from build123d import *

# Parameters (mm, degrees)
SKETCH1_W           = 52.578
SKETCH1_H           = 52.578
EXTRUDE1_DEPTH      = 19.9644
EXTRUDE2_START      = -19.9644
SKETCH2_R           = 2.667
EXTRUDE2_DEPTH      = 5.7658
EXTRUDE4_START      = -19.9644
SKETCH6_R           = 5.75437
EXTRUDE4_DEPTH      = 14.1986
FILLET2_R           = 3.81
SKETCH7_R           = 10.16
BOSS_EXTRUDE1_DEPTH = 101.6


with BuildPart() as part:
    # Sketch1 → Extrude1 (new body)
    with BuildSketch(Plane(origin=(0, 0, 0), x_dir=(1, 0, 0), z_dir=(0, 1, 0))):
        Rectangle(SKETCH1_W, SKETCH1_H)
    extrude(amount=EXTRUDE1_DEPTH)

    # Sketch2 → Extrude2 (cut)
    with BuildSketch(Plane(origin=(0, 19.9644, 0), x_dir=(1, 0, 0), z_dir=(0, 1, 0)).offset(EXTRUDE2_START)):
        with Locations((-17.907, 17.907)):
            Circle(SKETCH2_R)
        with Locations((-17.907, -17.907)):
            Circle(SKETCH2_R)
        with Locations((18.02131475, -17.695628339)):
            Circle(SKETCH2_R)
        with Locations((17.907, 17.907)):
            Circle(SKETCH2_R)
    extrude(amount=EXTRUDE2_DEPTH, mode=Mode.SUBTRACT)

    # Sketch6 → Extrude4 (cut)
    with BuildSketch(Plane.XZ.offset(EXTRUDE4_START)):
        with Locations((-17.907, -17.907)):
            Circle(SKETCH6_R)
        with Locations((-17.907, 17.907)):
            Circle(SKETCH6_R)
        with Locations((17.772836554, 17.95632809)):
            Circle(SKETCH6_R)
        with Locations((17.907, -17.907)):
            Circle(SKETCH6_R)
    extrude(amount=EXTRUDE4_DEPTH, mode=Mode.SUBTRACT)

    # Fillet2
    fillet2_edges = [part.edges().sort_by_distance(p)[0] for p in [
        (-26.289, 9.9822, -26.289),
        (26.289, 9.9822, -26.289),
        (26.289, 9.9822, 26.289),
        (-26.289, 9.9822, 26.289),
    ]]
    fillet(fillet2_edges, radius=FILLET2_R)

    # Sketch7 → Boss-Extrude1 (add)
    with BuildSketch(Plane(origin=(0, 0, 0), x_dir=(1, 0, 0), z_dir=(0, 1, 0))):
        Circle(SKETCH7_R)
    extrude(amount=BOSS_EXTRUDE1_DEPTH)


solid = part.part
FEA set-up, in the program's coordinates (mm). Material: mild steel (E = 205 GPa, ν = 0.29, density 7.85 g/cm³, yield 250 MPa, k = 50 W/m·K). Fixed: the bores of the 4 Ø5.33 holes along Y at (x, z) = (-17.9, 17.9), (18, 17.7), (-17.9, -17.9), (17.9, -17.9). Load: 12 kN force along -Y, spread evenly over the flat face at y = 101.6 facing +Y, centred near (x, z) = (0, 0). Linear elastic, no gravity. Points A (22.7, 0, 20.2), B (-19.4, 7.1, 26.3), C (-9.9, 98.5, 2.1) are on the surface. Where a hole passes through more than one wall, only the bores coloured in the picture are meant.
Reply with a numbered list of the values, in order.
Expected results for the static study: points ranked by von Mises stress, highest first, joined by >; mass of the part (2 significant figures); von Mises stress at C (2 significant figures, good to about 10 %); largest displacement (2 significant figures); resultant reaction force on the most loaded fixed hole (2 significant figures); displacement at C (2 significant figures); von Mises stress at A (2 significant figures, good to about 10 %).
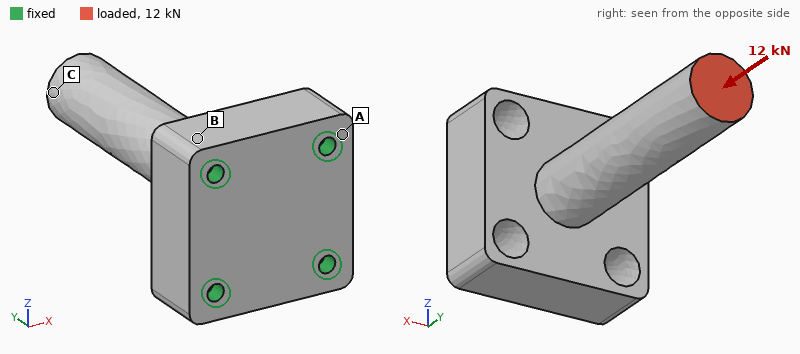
1. C > A > B
2. 590 g
3. 37 MPa
4. 20 µm
5. 3.3 kN
6. 19 µm
7. 21 MPa
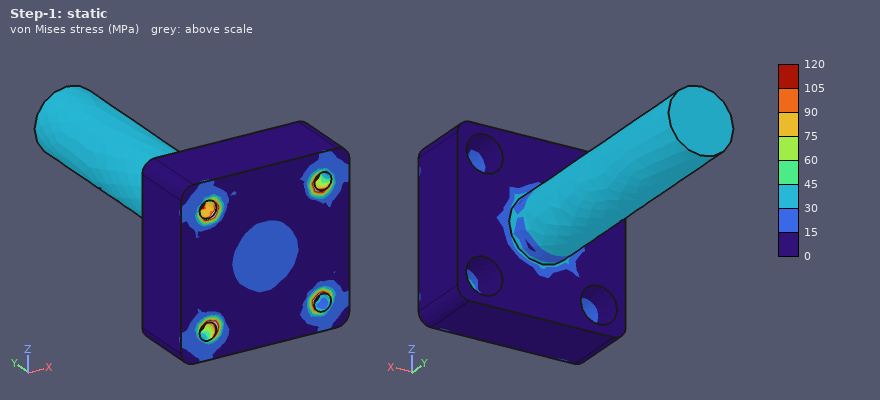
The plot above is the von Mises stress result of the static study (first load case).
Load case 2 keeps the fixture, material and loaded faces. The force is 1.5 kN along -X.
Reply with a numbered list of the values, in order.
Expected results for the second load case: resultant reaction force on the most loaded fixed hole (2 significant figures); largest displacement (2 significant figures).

1. 2.2 kN
2. 0.20 mm
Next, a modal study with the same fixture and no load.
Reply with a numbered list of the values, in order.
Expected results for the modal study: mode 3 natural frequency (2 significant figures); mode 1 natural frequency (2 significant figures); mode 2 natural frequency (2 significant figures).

1. 9400 Hz
2. 1800 Hz
3. 1800 Hz
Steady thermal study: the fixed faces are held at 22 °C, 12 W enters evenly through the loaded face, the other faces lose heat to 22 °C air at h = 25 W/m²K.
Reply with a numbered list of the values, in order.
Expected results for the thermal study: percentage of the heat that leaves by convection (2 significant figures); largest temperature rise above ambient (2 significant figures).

1. 34 %
2. 54 K
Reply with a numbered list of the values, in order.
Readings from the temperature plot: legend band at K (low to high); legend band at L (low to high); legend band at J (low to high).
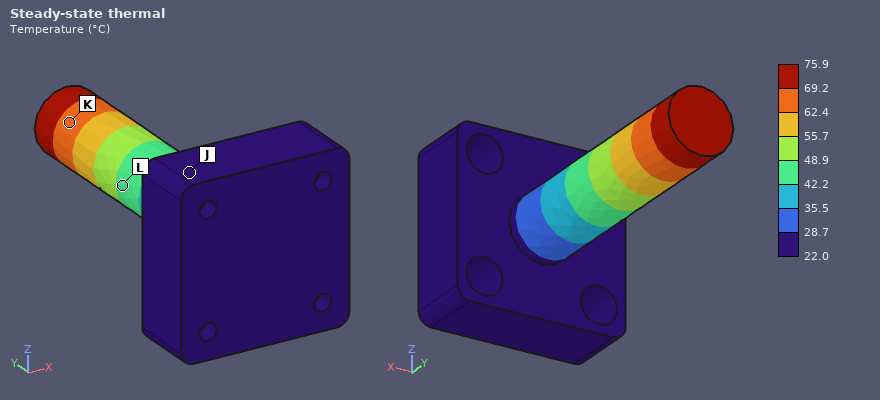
1. 62.4 to 69.2 °C
2. 42.2 to 48.9 °C
3. 22.0 to 28.7 °C
